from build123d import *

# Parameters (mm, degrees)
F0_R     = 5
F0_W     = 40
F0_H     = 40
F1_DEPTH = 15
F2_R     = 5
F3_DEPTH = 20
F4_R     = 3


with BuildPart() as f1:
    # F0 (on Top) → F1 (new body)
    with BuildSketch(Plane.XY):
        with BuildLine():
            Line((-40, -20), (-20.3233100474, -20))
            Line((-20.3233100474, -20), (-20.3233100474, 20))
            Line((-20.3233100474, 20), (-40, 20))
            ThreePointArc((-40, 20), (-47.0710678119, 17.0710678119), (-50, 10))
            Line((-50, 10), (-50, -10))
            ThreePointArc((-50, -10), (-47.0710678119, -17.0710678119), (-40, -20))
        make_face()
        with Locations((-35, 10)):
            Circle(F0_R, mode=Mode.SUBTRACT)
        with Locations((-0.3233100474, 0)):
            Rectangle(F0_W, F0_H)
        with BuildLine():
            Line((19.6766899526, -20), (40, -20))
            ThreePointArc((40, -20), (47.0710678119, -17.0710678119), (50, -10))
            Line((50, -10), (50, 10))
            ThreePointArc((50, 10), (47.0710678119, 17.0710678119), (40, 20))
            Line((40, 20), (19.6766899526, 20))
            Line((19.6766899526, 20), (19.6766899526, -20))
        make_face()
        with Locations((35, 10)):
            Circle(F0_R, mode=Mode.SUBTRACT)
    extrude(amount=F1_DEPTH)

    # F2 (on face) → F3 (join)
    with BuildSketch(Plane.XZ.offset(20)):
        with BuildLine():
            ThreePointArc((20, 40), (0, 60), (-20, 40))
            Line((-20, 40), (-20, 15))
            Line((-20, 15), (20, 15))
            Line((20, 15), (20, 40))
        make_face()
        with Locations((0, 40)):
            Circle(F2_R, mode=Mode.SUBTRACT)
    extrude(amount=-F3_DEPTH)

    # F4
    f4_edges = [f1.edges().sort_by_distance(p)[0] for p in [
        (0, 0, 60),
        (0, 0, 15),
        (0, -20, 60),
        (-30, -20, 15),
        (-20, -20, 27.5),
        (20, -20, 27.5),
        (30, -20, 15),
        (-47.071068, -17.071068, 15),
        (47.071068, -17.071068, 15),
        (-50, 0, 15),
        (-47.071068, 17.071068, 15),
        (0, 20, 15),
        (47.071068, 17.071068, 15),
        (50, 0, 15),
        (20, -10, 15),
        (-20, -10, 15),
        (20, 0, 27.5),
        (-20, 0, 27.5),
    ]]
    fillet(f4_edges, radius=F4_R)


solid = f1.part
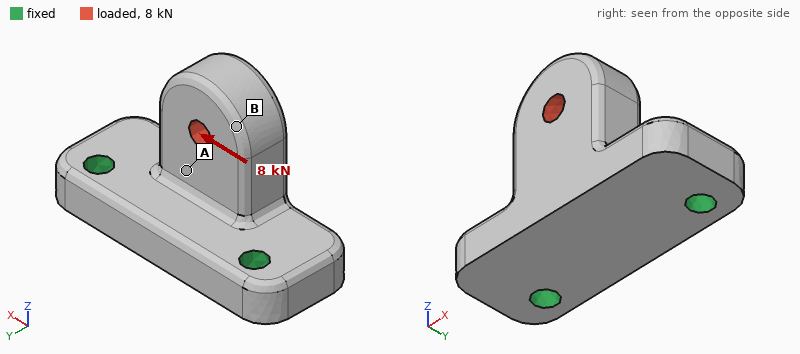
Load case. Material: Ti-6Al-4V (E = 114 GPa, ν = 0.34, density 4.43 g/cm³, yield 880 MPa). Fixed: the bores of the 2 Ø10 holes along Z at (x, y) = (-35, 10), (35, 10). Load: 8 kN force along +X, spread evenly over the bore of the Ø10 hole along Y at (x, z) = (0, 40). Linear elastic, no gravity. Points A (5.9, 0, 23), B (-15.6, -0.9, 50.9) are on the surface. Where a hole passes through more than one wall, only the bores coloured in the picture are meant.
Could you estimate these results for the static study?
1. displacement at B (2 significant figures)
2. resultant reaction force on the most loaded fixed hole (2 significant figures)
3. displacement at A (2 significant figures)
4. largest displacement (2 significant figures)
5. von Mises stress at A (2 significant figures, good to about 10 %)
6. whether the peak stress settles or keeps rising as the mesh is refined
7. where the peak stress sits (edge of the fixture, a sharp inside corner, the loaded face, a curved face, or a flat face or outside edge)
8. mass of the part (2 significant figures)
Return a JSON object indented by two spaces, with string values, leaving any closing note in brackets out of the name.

{
  "displacement at B": "42 µm",
  "resultant reaction force on the most loaded fixed hole": "6.2 kN",
  "displacement at A": "14 µm",
  "largest displacement": "46 µm",
  "von Mises stress at A": "32 MPa",
  "whether the peak stress settles or keeps rising as the mesh is refined": "keeps rising",
  "where the peak stress sits": "a sharp inside corner",
  "mass of the part": "380 g"
}
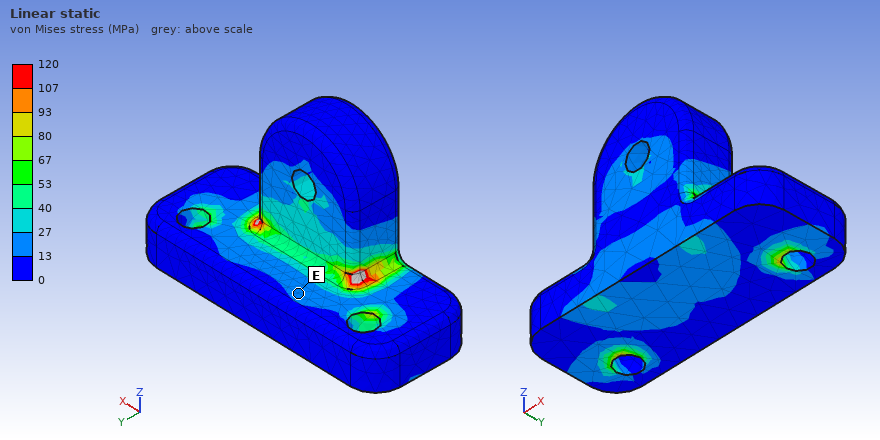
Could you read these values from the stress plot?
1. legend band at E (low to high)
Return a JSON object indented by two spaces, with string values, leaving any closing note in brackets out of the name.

{
  "legend band at E": "13 to 27 MPa"
}
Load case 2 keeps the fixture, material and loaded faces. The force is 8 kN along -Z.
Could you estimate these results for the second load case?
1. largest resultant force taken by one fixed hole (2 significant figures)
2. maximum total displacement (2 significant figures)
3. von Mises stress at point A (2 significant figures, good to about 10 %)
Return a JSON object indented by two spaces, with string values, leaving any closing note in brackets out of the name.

{
  "largest resultant force taken by one fixed hole": "4.0 kN",
  "maximum total displacement": "62 µm",
  "von Mises stress at point A": "11 MPa"
}
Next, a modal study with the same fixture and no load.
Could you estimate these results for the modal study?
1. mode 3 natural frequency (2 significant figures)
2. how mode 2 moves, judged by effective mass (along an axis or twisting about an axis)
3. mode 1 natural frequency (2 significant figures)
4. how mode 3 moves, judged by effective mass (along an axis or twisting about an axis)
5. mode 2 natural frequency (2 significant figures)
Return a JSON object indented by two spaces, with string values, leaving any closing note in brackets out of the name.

{
  "mode 3 natural frequency": "8400 Hz",
  "how mode 2 moves, judged by effective mass": "along X",
  "mode 1 natural frequency": "3500 Hz",
  "how mode 3 moves, judged by effective mass": "along Z",
  "mode 2 natural frequency": "7000 Hz"
}
